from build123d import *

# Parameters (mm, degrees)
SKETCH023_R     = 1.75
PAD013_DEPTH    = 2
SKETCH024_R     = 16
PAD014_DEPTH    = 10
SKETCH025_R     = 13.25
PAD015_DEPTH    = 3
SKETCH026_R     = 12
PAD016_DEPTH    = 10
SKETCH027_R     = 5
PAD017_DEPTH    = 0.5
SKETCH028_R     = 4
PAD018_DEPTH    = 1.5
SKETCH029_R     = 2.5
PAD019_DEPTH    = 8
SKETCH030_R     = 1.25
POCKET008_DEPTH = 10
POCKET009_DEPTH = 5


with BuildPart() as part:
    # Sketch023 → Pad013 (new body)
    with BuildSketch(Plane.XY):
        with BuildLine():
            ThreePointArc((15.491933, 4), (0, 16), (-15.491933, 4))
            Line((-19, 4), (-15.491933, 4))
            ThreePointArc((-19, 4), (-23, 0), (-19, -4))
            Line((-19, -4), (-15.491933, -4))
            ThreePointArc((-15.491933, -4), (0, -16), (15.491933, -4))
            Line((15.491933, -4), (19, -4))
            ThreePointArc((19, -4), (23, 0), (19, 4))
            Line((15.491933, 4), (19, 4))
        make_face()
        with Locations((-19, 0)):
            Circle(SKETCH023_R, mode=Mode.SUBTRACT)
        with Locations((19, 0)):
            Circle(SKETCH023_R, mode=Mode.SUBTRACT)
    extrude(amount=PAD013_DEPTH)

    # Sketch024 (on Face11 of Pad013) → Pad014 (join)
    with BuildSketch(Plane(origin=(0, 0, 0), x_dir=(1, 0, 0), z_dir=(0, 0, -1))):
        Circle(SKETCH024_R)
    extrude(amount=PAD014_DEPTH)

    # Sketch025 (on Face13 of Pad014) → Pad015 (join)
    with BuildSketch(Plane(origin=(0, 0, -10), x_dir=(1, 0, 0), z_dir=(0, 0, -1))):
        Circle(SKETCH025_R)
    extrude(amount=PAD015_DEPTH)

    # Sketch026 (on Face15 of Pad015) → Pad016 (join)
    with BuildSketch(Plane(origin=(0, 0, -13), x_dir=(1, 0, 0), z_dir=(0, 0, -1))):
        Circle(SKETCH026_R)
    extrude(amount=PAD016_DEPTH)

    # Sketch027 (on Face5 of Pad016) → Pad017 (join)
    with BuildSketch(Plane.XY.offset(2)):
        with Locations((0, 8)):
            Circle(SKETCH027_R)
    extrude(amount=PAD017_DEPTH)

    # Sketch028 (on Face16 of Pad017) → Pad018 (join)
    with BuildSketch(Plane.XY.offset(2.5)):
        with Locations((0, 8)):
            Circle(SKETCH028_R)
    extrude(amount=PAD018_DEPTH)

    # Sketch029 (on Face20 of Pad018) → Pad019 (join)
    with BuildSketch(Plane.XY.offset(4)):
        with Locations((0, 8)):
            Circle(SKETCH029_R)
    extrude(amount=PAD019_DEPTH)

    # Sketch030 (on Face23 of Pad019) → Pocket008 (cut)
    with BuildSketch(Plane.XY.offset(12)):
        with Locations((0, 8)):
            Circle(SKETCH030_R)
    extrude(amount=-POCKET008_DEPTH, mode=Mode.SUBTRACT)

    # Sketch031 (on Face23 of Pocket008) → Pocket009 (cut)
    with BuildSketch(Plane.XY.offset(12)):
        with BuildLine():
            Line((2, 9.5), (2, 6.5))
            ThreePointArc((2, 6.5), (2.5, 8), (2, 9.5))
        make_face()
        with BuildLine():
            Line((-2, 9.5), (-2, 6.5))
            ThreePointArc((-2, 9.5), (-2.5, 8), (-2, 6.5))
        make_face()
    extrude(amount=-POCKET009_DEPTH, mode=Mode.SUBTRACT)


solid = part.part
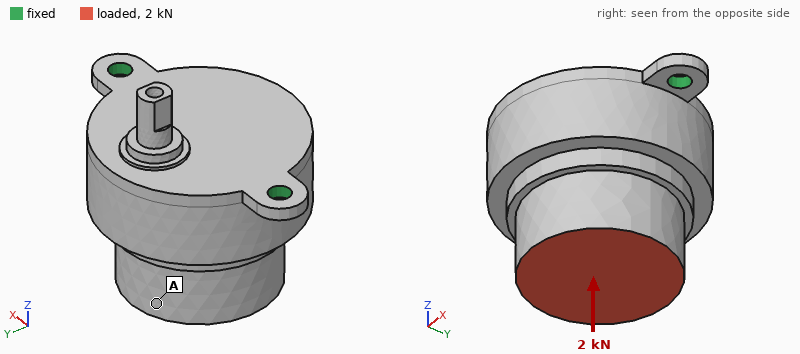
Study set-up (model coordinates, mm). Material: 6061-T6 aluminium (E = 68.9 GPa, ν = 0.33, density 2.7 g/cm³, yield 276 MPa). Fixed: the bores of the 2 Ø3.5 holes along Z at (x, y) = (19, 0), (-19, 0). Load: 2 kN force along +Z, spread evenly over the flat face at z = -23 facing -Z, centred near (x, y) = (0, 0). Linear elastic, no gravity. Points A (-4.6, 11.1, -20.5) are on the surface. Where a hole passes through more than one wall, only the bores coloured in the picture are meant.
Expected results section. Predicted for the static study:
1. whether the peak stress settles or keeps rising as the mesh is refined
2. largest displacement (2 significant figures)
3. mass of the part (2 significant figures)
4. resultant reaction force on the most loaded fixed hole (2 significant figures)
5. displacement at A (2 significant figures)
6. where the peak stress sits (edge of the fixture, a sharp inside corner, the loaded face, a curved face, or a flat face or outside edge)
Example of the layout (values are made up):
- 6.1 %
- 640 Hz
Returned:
- keeps rising
- 18 µm
- 44 g
- 1.2 kN
- 18 µm
- edge of the fixture
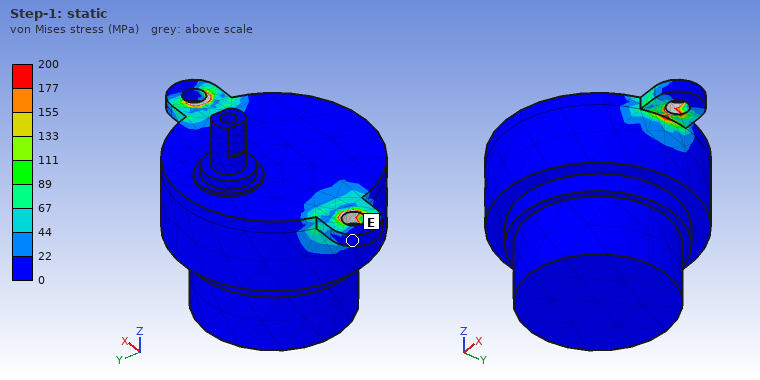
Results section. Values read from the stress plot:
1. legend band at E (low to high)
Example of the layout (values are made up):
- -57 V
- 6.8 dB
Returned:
- 0 to 22 MPa
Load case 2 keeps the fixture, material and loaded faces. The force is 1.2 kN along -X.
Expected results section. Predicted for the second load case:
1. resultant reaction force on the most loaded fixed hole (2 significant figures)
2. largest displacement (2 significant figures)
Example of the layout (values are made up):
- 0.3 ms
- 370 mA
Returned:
- 1.1 kN
- 26 µm
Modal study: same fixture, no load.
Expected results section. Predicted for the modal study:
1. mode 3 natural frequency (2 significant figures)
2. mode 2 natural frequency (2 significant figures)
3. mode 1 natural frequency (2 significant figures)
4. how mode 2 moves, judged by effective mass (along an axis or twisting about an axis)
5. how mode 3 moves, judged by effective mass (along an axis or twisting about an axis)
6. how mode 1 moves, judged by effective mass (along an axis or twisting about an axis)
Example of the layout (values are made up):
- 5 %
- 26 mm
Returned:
- 9600 Hz
- 8300 Hz
- 1300 Hz
- along Z
- along X
- along Y
